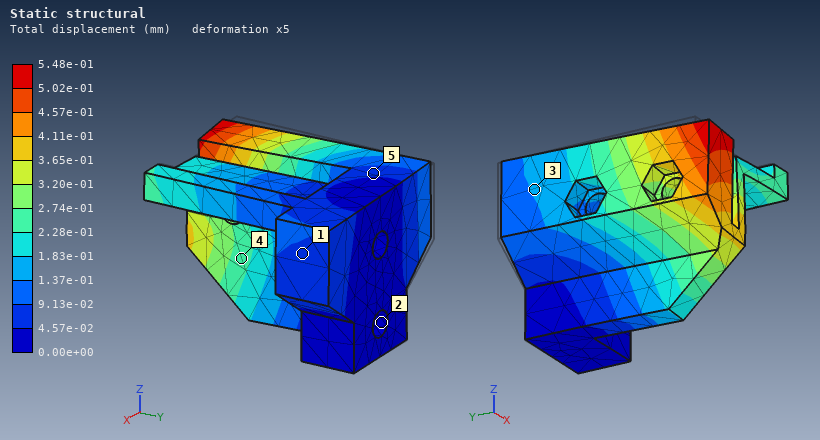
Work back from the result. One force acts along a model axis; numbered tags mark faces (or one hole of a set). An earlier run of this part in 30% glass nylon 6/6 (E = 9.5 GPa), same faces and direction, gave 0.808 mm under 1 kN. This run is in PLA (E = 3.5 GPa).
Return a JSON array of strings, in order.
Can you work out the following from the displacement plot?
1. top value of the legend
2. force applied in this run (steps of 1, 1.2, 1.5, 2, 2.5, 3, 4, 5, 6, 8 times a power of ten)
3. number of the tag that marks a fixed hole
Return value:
["5.48e-01 mm", "250 N", "2"]
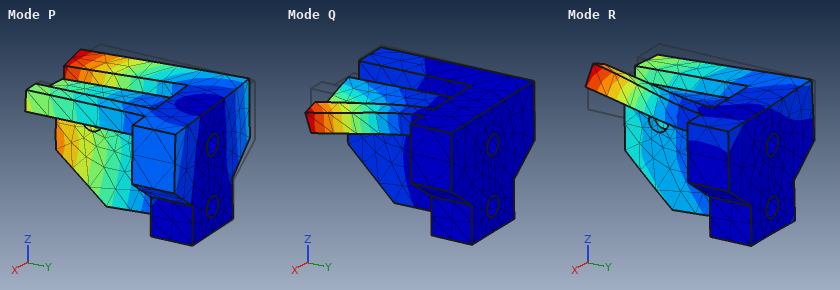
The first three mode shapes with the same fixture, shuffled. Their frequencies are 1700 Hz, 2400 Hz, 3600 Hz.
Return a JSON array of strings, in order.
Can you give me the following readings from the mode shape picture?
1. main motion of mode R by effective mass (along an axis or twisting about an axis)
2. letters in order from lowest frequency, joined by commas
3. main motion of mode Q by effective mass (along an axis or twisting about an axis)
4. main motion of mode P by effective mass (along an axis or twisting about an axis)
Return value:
["along Z", "P, Q, R", "along Z", "along X"]
